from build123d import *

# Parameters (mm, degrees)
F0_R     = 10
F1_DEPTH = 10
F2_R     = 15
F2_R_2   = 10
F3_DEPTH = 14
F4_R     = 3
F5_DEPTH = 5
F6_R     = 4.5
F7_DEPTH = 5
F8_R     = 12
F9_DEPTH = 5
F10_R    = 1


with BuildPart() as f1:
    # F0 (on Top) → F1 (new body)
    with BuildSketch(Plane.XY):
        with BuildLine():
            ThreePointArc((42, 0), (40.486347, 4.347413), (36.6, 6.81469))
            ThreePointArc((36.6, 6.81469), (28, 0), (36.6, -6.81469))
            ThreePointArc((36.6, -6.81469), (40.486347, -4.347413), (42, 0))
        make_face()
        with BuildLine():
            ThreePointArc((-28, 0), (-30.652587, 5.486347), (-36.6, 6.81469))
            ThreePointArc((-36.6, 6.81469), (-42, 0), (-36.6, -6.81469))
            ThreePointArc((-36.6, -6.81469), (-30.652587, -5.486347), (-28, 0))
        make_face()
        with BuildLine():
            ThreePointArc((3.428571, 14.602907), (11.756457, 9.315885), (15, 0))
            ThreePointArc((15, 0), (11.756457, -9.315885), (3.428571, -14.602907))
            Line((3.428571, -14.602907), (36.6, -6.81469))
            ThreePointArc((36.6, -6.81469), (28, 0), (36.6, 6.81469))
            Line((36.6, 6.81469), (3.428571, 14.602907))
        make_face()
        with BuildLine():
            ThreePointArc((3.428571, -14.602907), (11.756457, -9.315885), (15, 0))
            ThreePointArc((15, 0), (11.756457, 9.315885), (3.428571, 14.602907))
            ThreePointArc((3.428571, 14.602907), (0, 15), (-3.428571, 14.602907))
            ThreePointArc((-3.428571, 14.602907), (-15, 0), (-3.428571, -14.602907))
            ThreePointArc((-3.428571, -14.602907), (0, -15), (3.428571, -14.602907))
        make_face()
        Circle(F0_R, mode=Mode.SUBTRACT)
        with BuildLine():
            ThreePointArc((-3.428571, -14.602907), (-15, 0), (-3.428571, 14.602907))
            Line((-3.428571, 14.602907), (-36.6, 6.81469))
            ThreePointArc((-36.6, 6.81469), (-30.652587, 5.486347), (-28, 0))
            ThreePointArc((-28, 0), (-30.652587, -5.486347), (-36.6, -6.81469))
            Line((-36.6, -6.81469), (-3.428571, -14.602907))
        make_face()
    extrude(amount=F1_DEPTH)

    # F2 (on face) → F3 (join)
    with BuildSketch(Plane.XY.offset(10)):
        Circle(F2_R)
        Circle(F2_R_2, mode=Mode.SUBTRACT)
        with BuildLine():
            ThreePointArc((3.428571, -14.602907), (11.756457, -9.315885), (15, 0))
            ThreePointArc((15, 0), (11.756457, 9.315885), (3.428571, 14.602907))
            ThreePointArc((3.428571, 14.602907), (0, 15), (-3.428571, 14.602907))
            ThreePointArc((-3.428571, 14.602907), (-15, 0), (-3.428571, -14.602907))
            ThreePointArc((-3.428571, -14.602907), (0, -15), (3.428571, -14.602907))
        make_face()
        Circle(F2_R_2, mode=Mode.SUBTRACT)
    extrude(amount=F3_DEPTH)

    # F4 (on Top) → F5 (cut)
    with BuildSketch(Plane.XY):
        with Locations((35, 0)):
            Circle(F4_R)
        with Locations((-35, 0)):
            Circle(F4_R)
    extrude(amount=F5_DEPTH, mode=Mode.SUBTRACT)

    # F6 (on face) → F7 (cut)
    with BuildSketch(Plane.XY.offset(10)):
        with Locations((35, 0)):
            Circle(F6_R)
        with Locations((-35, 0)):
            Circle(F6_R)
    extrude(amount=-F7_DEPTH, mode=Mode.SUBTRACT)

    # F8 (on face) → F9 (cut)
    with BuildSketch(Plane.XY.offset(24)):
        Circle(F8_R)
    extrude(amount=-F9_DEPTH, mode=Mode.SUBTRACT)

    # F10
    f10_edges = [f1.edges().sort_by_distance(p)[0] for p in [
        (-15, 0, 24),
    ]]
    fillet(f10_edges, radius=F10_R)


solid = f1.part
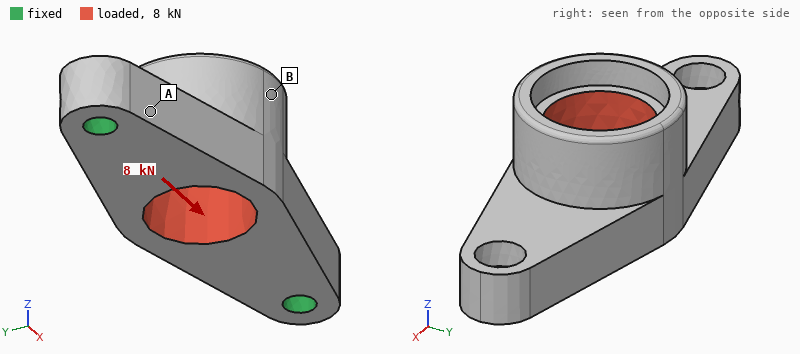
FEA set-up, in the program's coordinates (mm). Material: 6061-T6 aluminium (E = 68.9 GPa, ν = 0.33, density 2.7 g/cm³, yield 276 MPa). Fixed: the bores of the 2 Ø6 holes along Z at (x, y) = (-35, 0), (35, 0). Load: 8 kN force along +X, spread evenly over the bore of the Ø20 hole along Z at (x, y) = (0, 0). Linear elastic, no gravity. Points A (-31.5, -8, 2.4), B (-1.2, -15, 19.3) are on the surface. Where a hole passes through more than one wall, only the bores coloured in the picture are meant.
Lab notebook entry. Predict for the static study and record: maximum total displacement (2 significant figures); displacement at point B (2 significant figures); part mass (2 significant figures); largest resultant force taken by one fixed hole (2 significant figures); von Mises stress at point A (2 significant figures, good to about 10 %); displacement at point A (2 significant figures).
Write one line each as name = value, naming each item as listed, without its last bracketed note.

maximum total displacement = 18 µm
displacement at point B = 16 µm
part mass = 49 g
largest resultant force taken by one fixed hole = 4.1 kN
von Mises stress at point A = 18 MPa
displacement at point A = 4.4 µm
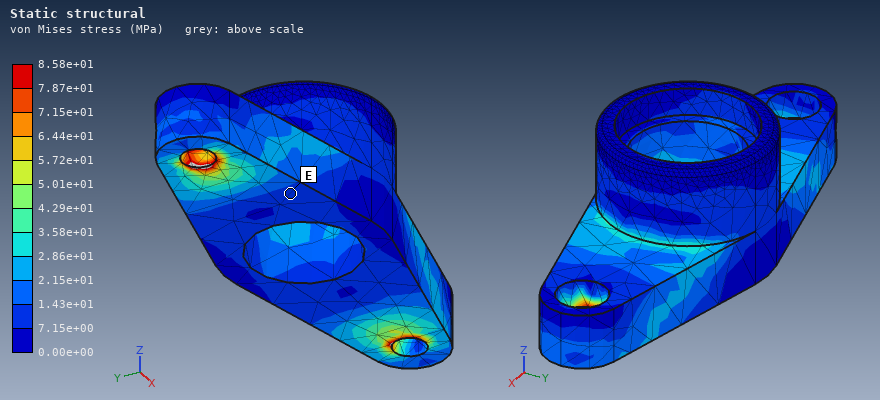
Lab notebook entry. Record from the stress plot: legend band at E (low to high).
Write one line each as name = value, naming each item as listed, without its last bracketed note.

legend band at E = 7.15e+00 to 1.43e+01 MPa
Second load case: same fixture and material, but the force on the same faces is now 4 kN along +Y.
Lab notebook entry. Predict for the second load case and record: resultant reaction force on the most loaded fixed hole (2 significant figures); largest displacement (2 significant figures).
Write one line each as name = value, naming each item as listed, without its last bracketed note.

resultant reaction force on the most loaded fixed hole = 2.0 kN
largest displacement = 0.11 mm
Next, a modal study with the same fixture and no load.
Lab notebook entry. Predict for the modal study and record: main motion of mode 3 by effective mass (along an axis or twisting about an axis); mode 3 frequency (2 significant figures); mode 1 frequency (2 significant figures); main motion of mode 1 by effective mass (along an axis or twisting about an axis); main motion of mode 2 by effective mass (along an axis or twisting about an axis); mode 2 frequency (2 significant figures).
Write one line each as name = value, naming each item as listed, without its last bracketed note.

main motion of mode 3 by effective mass = along Y
mode 3 frequency = 12 kHz
mode 1 frequency = 5500 Hz
main motion of mode 1 by effective mass = along Y
main motion of mode 2 by effective mass = along Z
mode 2 frequency = 6800 Hz
